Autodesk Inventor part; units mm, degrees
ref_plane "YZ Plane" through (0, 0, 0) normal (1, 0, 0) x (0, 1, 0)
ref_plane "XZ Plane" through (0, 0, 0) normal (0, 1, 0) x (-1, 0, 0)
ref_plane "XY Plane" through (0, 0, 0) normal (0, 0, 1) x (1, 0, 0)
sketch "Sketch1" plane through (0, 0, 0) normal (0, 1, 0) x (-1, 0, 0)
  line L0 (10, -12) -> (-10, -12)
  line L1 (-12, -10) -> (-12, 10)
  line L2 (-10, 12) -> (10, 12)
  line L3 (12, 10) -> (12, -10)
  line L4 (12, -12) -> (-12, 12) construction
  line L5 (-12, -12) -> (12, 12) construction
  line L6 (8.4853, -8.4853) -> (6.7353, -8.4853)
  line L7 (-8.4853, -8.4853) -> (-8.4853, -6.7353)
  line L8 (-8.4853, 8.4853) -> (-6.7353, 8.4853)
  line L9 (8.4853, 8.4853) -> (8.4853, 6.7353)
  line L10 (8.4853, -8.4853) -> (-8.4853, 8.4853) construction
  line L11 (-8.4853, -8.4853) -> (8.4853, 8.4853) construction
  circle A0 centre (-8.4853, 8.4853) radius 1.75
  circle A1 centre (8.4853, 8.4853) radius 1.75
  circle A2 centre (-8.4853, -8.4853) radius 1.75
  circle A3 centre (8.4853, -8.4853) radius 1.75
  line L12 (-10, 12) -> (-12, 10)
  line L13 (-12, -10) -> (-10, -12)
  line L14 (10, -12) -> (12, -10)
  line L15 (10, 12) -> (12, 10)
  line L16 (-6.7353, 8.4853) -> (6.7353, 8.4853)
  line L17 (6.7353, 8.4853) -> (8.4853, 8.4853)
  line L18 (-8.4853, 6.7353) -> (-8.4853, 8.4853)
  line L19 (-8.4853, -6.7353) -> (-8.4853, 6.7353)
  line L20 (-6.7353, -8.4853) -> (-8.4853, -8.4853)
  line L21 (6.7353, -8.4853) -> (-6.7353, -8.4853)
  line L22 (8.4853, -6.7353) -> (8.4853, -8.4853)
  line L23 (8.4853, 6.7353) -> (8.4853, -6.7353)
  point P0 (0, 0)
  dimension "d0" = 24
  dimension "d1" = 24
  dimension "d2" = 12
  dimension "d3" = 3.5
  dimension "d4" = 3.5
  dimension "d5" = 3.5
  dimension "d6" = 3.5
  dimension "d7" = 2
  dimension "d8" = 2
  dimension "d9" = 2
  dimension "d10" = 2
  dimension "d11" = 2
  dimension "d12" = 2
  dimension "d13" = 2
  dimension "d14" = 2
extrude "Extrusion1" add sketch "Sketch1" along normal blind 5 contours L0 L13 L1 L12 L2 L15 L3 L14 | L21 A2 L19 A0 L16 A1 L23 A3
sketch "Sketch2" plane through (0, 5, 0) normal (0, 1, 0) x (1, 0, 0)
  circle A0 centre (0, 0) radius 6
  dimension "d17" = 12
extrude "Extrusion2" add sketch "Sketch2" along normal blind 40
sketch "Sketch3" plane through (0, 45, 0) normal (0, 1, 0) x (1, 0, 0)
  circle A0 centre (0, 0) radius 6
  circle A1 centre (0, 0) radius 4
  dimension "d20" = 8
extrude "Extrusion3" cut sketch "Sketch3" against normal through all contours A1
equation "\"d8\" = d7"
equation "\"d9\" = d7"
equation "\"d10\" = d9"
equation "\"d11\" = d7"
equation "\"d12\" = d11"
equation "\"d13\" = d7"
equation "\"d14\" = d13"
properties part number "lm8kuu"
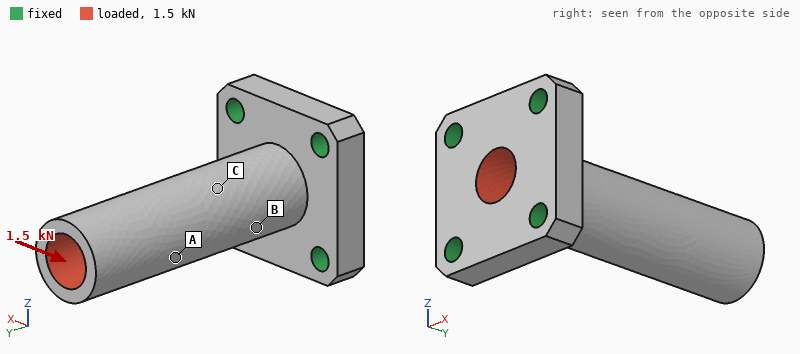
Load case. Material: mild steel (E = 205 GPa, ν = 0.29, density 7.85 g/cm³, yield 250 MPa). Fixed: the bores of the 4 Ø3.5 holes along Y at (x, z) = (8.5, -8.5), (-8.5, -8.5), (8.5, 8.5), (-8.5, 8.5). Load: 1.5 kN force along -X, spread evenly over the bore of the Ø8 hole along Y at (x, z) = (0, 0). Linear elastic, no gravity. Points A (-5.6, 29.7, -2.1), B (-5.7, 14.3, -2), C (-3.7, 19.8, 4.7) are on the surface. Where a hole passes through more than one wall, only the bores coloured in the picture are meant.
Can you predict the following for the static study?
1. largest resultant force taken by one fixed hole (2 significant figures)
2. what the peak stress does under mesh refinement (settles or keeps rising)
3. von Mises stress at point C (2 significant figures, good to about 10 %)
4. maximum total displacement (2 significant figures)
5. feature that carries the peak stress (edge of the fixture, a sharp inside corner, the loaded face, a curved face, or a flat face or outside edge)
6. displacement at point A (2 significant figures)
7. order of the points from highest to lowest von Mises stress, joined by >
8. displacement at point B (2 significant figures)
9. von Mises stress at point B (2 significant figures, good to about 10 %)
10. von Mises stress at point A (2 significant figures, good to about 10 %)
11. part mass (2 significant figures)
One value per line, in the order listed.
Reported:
1.1 kN
keeps rising
57 MPa
0.11 mm
a sharp inside corner
0.065 mm
B > C > A
0.023 mm
110 MPa
28 MPa
39 g
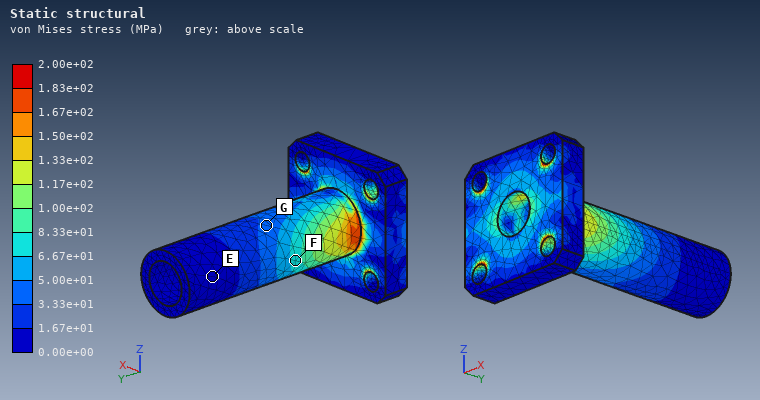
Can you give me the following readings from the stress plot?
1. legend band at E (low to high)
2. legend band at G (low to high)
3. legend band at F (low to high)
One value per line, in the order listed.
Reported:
0.00e+00 to 1.67e+01 MPa
3.33e+01 to 5.00e+01 MPa
6.67e+01 to 8.33e+01 MPa
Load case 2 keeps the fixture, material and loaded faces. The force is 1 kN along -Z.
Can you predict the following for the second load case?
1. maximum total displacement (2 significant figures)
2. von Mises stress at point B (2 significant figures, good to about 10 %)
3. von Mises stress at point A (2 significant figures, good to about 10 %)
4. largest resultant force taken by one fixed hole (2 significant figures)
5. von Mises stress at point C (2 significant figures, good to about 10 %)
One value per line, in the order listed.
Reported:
74 µm
39 MPa
16 MPa
760 N
44 MPa
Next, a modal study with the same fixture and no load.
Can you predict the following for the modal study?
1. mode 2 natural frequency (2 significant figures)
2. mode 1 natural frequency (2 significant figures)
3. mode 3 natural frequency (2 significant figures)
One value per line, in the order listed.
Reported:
4800 Hz
4800 Hz
19 kHz
